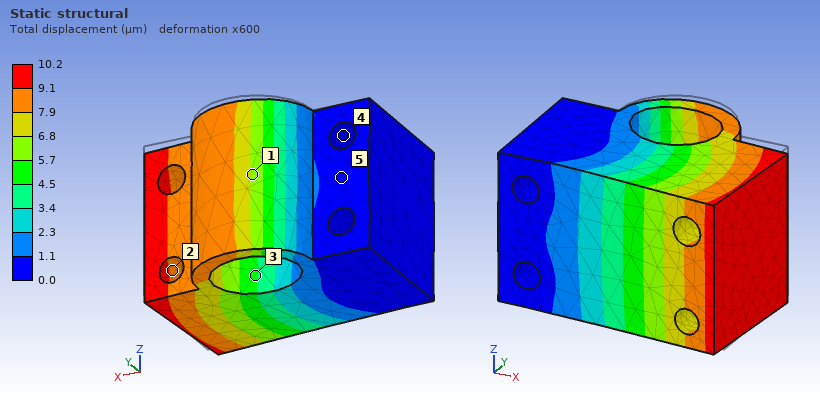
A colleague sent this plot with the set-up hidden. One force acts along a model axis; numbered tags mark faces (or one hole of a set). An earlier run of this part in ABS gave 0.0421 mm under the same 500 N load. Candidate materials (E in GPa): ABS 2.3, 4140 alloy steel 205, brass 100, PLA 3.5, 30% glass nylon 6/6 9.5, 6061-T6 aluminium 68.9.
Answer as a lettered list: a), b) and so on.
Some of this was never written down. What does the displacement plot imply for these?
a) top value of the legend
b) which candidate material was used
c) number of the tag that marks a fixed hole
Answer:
a) 10.2 µm
b) 30% glass nylon 6/6
c) 4
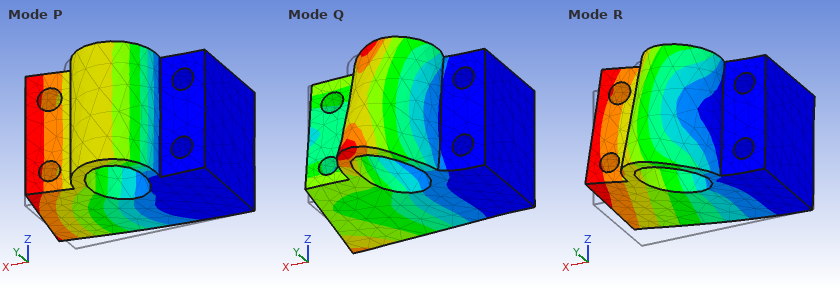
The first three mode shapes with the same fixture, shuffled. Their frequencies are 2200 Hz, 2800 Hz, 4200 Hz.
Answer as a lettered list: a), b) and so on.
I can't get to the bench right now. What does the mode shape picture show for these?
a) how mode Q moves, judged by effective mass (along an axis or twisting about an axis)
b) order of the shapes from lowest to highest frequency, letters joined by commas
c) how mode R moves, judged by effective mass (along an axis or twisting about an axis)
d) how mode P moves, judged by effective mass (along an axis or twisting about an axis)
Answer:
a) twisting about X
b) P, R, Q
c) along Z
d) along Y
